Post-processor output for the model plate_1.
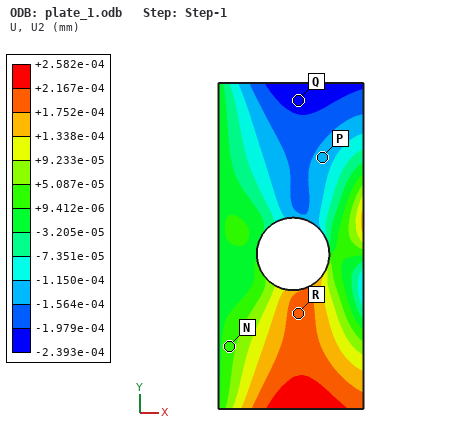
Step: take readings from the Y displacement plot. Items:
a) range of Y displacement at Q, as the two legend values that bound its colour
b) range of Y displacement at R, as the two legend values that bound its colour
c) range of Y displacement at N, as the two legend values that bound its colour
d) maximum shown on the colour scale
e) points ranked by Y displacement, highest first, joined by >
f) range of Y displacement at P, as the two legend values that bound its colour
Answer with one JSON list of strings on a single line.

["-2.393e-04 to -1.979e-04 mm", "+1.752e-04 to +2.167e-04 mm", "+9.412e-06 to +5.087e-05 mm", "+2.582e-04 mm", "R > N > P > Q", "-1.564e-04 to -1.150e-04 mm"]
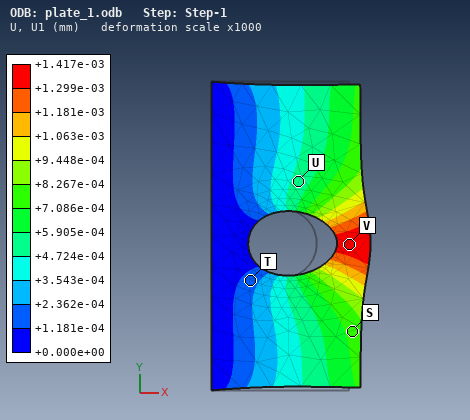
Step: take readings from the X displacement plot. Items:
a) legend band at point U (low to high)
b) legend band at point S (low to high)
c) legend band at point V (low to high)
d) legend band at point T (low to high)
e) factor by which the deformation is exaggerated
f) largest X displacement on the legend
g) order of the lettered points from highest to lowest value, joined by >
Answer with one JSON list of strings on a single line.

["+4.724e-04 to +5.905e-04 mm", "+7.086e-04 to +8.267e-04 mm", "+1.299e-03 to +1.417e-03 mm", "+1.181e-04 to +2.362e-04 mm", "1000", "+1.417e-03 mm", "V > S > U > T"]
